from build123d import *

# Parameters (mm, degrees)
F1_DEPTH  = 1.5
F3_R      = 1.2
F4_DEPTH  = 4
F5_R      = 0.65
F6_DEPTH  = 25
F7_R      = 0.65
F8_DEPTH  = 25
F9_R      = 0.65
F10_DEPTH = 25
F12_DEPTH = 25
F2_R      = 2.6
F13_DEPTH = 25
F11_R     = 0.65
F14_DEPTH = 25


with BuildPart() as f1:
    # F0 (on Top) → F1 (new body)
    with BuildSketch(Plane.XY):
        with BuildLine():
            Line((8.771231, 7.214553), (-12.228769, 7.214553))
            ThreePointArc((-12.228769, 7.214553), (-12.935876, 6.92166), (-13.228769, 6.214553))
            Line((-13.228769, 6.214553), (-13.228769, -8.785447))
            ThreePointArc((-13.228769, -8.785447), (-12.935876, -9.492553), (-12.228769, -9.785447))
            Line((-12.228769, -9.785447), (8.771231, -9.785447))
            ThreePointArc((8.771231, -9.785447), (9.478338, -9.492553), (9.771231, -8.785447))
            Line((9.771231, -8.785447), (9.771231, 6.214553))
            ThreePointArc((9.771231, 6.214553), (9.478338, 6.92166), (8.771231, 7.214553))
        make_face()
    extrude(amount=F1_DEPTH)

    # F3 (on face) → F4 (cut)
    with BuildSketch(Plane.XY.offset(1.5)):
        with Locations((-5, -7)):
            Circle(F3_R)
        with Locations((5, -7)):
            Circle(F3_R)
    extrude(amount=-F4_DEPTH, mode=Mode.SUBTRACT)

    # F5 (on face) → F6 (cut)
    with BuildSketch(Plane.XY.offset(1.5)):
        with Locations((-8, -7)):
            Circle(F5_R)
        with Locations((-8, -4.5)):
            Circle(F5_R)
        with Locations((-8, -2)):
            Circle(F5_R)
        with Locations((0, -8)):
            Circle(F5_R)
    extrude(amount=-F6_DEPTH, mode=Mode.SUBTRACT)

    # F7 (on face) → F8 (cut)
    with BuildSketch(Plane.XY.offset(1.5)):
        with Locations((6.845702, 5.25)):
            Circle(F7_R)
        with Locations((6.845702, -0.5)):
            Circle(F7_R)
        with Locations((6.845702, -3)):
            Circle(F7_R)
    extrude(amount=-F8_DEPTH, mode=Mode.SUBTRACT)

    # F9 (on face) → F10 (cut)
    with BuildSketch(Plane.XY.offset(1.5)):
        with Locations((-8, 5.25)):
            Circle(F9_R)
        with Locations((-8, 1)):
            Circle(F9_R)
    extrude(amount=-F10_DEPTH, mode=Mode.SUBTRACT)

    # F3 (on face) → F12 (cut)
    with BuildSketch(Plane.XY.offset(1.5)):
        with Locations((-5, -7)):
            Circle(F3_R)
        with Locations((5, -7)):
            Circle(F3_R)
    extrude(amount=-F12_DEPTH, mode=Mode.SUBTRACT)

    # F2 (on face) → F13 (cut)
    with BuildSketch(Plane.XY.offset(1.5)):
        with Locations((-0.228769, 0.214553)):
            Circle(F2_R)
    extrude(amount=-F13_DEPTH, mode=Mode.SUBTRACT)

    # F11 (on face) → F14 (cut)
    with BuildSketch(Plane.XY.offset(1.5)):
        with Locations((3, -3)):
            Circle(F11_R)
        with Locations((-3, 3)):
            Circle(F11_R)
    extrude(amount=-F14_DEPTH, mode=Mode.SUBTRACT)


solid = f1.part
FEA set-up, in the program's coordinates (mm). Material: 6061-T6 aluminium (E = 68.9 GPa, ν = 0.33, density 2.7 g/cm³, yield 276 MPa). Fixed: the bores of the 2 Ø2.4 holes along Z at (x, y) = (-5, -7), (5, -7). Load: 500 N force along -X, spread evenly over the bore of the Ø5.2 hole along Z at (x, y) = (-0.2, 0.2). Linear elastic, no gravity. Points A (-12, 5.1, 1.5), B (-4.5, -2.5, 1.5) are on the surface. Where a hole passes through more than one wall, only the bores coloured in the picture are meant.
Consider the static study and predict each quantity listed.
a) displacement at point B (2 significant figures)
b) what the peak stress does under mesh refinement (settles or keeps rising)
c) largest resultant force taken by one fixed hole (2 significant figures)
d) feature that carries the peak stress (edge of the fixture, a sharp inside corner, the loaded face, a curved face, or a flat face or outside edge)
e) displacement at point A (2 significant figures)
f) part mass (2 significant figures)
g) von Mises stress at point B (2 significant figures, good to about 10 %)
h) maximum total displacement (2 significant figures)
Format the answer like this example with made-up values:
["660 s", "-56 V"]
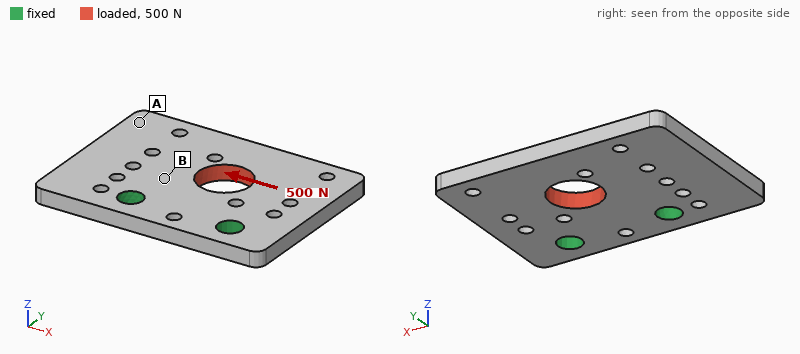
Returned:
["5.3 µm", "keeps rising", "370 N", "edge of the fixture", "17 µm", "1.4 g", "37 MPa", "19 µm"]
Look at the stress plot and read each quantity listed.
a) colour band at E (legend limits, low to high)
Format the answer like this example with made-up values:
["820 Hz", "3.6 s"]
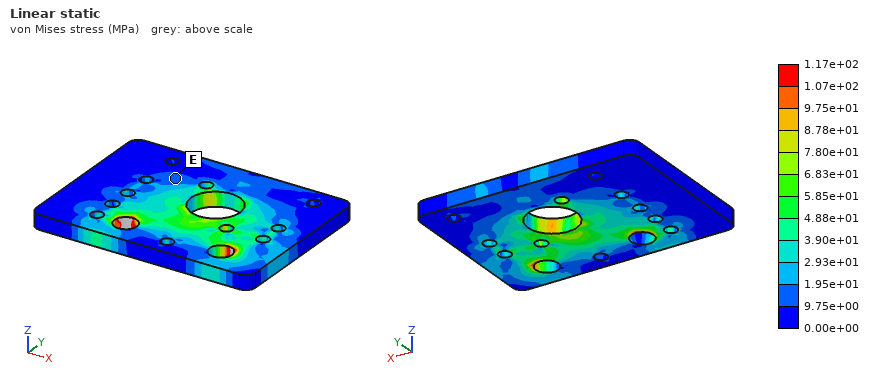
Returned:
["9.75e+00 to 1.95e+01 MPa"]
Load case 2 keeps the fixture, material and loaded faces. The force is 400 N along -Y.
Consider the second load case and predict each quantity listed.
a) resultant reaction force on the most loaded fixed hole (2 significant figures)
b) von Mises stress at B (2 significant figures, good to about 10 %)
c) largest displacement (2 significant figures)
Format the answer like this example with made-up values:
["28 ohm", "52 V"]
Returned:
["220 N", "25 MPa", "4.5 µm"]
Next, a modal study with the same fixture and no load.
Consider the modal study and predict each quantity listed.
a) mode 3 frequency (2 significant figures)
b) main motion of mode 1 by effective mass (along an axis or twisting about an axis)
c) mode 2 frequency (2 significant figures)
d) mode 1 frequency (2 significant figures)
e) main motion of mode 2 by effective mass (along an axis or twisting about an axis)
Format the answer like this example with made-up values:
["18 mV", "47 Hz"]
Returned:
["17 kHz", "along Z", "8800 Hz", "5800 Hz", "twisting about Y"]
